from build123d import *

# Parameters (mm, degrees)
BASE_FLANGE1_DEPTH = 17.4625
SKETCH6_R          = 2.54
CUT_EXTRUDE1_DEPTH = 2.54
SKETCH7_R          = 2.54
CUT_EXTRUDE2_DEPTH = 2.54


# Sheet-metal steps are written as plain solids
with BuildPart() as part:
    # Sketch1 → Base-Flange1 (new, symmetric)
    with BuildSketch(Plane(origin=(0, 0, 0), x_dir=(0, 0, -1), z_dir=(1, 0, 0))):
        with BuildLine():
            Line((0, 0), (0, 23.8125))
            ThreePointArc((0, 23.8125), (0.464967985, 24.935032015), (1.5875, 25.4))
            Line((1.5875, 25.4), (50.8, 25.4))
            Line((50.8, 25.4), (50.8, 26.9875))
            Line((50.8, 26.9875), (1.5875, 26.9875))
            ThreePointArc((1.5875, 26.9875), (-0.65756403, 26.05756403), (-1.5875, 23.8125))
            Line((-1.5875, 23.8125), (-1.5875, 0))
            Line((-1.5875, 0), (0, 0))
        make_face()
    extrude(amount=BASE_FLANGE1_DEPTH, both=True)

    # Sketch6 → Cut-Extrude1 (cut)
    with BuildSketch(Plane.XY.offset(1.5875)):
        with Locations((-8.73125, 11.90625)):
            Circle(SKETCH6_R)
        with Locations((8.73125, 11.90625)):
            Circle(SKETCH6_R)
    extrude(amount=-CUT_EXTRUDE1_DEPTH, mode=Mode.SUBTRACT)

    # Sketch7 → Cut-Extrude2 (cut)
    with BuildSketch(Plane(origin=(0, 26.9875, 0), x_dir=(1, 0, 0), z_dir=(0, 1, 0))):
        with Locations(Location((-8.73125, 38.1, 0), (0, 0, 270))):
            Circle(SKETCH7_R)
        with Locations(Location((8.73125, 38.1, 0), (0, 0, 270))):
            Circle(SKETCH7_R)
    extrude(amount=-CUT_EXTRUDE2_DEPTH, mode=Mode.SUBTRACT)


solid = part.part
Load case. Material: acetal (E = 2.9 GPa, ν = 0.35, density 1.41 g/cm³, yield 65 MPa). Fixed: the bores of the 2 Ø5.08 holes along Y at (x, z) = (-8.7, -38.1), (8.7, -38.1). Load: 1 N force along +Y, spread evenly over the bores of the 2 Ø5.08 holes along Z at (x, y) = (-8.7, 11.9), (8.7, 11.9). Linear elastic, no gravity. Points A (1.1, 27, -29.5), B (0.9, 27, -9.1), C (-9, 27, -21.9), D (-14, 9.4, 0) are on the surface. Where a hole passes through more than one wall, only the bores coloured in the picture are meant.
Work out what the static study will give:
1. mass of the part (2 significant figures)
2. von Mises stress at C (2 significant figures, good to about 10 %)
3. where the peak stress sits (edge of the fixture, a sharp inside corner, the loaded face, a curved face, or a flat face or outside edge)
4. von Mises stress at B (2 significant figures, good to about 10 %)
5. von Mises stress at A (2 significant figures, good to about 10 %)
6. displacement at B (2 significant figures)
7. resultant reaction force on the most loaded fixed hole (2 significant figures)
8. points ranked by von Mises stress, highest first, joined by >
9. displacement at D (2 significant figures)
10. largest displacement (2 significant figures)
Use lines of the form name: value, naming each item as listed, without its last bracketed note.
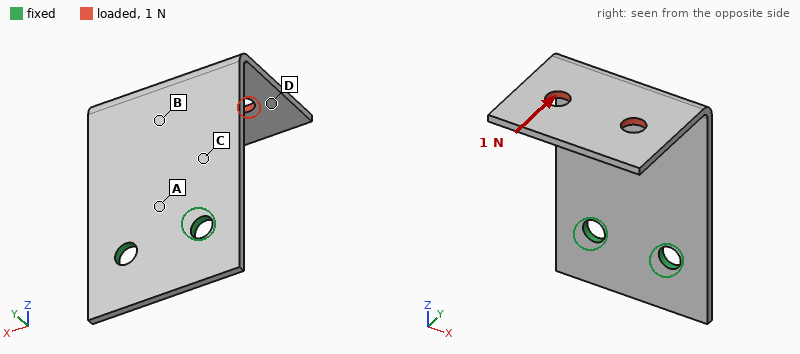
mass of the part: 5.8 g
von Mises stress at C: 1.4 MPa
where the peak stress sits: a flat face or outside edge
von Mises stress at B: 0.61 MPa
von Mises stress at A: 1.9 MPa
displacement at B: 0.30 mm
resultant reaction force on the most loaded fixed hole: 0.50 N
points ranked by von Mises stress, highest first, joined by >: A > C > B > D
displacement at D: 0.57 mm
largest displacement: 0.71 mm
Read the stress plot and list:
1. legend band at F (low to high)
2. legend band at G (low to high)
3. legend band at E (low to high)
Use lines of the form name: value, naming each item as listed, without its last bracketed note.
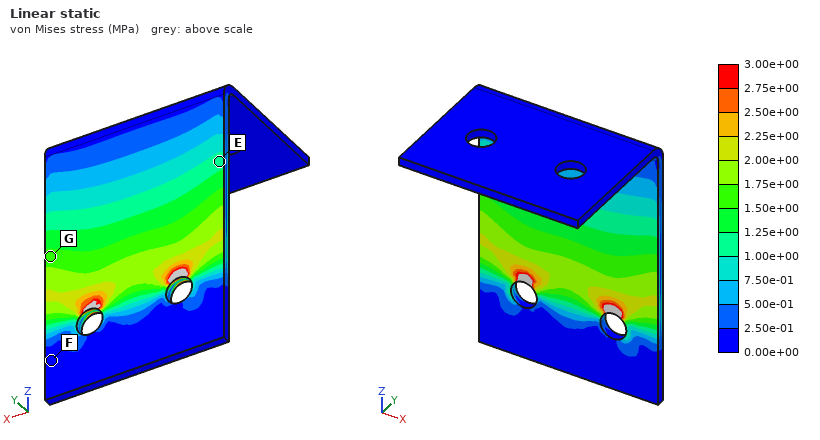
legend band at F: 0.00e+00 to 2.50e-01 MPa
legend band at G: 1.50e+00 to 1.75e+00 MPa
legend band at E: 1.00e+00 to 1.25e+00 MPa
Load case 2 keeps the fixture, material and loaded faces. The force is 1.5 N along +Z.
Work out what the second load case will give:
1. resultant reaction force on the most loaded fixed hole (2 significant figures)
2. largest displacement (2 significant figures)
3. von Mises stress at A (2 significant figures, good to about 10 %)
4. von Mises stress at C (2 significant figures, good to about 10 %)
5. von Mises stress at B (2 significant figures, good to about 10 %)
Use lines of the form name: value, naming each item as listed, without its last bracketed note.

resultant reaction force on the most loaded fixed hole: 0.76 N
largest displacement: 0.79 mm
von Mises stress at A: 1.3 MPa
von Mises stress at C: 1.3 MPa
von Mises stress at B: 1.3 MPa
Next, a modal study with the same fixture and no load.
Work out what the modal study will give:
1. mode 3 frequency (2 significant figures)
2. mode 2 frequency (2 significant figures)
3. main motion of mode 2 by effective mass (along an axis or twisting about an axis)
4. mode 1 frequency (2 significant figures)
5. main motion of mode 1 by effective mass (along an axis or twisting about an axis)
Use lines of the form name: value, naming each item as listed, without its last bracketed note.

mode 3 frequency: 400 Hz
mode 2 frequency: 260 Hz
main motion of mode 2 by effective mass: along X
mode 1 frequency: 120 Hz
main motion of mode 1 by effective mass: along Y
